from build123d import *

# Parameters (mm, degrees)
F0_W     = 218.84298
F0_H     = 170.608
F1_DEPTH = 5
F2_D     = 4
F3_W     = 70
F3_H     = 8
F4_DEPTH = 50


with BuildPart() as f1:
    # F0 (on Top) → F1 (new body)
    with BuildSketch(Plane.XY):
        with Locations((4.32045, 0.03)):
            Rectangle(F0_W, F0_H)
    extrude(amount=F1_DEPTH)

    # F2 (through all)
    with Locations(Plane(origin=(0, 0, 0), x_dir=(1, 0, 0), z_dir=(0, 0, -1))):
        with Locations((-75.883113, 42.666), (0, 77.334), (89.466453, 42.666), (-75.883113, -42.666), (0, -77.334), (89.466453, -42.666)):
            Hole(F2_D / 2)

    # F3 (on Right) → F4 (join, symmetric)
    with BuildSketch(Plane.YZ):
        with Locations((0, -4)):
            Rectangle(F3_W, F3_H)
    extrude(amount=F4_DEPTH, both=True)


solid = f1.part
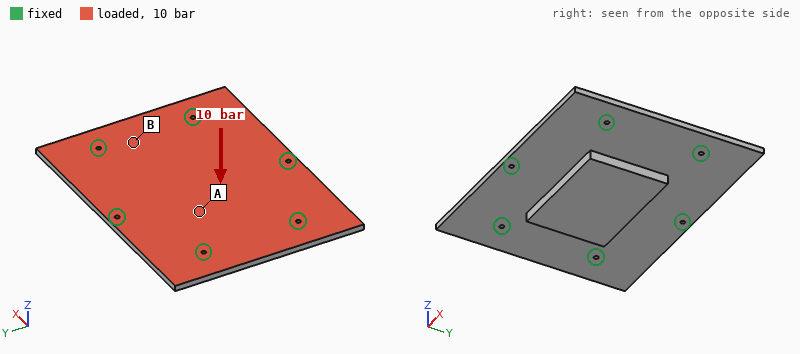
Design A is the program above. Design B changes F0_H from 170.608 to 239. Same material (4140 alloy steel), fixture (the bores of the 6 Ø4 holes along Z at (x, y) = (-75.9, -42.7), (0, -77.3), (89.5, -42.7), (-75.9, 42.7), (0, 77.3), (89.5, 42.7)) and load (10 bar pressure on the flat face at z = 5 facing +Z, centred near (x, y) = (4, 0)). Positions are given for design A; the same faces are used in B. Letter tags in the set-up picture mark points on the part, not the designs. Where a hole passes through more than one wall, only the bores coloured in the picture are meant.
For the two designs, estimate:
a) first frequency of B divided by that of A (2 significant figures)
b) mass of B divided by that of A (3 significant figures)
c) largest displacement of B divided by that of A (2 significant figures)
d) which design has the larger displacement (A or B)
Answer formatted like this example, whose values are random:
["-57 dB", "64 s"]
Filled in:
["0.61", "1.31", "6.9", "B"]
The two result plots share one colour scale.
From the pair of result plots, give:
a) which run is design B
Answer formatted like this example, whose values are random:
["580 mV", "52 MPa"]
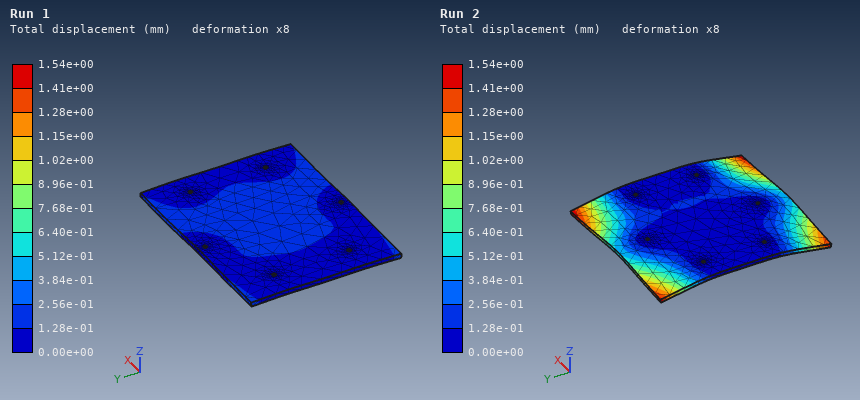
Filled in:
["Run 2"]
